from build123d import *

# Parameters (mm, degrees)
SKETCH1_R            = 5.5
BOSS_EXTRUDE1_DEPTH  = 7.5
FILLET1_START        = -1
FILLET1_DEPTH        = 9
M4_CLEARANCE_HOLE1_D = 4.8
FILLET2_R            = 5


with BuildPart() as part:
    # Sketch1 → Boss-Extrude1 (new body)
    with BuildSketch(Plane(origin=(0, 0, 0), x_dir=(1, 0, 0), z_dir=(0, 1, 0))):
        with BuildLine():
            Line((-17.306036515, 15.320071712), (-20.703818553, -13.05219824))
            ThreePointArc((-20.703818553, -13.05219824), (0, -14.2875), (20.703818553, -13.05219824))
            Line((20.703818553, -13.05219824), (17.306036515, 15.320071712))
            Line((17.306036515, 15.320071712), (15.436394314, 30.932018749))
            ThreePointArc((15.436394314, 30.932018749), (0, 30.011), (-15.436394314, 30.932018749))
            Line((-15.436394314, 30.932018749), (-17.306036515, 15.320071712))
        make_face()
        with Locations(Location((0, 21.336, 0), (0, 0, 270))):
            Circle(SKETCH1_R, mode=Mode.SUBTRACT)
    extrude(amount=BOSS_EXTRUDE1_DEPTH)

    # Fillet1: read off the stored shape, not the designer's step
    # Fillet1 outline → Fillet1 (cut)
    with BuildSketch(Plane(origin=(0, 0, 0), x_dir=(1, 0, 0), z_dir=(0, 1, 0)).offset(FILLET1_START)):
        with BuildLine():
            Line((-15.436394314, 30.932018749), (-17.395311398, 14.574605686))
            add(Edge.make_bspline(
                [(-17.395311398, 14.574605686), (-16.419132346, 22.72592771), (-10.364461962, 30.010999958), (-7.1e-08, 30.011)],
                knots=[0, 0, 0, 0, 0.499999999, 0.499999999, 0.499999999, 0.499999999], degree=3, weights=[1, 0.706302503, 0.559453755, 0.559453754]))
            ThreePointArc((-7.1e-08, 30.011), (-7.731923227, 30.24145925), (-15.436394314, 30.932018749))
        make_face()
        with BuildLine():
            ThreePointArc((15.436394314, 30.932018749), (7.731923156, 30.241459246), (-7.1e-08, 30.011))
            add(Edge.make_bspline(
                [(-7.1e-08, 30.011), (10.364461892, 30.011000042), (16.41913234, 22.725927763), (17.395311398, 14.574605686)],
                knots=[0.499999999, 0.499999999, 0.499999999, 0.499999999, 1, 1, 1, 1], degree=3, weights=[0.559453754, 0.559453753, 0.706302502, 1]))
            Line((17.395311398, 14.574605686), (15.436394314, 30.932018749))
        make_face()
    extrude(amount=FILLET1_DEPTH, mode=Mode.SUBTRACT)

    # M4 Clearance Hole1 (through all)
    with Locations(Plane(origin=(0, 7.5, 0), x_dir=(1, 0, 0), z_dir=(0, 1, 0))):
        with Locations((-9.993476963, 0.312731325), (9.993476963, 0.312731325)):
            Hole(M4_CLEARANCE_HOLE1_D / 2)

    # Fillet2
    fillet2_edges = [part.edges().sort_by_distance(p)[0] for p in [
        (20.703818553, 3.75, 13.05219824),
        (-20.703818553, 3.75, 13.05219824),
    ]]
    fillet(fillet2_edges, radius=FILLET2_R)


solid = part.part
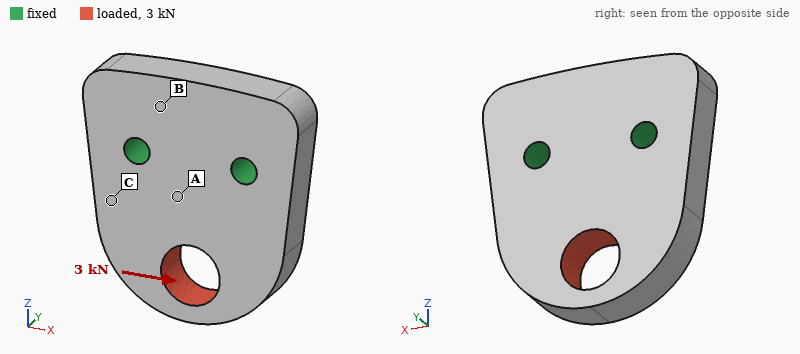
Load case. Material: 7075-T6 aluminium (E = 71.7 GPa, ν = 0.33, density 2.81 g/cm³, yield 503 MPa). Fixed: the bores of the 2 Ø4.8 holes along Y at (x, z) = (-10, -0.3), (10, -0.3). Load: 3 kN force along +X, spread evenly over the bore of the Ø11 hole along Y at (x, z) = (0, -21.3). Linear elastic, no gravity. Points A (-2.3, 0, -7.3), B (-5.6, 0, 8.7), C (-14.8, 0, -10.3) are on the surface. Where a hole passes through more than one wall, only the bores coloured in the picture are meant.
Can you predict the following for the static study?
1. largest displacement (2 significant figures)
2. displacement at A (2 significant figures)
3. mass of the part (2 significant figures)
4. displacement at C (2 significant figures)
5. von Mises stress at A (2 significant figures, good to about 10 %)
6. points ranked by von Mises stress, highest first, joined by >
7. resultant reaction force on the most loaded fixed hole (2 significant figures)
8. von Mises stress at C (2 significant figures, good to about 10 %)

28 µm
4.2 µm
29 g
8.5 µm
35 MPa
A > C > B
3.0 kN
20 MPa
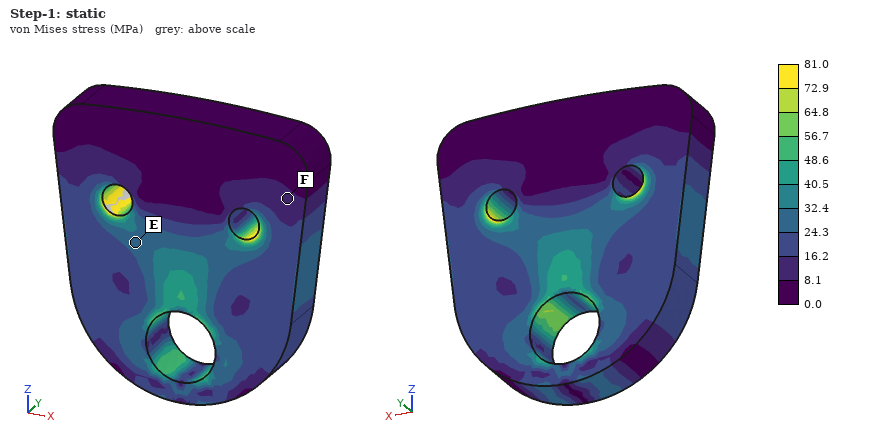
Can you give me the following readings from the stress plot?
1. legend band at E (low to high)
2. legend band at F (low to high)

24.3 to 32.4 MPa
8.1 to 16.2 MPa
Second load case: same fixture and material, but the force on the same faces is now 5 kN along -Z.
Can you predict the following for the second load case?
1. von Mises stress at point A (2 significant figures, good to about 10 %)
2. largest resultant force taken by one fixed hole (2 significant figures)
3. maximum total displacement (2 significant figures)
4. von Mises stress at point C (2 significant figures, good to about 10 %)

16 MPa
2.6 kN
18 µm
14 MPa
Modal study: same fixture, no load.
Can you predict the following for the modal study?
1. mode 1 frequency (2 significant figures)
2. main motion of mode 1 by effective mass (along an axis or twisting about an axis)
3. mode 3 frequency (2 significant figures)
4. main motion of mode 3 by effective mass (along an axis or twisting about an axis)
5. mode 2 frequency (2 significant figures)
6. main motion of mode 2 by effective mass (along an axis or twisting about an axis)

9200 Hz
along Y
22 kHz
along X
17 kHz
twisting about Z
